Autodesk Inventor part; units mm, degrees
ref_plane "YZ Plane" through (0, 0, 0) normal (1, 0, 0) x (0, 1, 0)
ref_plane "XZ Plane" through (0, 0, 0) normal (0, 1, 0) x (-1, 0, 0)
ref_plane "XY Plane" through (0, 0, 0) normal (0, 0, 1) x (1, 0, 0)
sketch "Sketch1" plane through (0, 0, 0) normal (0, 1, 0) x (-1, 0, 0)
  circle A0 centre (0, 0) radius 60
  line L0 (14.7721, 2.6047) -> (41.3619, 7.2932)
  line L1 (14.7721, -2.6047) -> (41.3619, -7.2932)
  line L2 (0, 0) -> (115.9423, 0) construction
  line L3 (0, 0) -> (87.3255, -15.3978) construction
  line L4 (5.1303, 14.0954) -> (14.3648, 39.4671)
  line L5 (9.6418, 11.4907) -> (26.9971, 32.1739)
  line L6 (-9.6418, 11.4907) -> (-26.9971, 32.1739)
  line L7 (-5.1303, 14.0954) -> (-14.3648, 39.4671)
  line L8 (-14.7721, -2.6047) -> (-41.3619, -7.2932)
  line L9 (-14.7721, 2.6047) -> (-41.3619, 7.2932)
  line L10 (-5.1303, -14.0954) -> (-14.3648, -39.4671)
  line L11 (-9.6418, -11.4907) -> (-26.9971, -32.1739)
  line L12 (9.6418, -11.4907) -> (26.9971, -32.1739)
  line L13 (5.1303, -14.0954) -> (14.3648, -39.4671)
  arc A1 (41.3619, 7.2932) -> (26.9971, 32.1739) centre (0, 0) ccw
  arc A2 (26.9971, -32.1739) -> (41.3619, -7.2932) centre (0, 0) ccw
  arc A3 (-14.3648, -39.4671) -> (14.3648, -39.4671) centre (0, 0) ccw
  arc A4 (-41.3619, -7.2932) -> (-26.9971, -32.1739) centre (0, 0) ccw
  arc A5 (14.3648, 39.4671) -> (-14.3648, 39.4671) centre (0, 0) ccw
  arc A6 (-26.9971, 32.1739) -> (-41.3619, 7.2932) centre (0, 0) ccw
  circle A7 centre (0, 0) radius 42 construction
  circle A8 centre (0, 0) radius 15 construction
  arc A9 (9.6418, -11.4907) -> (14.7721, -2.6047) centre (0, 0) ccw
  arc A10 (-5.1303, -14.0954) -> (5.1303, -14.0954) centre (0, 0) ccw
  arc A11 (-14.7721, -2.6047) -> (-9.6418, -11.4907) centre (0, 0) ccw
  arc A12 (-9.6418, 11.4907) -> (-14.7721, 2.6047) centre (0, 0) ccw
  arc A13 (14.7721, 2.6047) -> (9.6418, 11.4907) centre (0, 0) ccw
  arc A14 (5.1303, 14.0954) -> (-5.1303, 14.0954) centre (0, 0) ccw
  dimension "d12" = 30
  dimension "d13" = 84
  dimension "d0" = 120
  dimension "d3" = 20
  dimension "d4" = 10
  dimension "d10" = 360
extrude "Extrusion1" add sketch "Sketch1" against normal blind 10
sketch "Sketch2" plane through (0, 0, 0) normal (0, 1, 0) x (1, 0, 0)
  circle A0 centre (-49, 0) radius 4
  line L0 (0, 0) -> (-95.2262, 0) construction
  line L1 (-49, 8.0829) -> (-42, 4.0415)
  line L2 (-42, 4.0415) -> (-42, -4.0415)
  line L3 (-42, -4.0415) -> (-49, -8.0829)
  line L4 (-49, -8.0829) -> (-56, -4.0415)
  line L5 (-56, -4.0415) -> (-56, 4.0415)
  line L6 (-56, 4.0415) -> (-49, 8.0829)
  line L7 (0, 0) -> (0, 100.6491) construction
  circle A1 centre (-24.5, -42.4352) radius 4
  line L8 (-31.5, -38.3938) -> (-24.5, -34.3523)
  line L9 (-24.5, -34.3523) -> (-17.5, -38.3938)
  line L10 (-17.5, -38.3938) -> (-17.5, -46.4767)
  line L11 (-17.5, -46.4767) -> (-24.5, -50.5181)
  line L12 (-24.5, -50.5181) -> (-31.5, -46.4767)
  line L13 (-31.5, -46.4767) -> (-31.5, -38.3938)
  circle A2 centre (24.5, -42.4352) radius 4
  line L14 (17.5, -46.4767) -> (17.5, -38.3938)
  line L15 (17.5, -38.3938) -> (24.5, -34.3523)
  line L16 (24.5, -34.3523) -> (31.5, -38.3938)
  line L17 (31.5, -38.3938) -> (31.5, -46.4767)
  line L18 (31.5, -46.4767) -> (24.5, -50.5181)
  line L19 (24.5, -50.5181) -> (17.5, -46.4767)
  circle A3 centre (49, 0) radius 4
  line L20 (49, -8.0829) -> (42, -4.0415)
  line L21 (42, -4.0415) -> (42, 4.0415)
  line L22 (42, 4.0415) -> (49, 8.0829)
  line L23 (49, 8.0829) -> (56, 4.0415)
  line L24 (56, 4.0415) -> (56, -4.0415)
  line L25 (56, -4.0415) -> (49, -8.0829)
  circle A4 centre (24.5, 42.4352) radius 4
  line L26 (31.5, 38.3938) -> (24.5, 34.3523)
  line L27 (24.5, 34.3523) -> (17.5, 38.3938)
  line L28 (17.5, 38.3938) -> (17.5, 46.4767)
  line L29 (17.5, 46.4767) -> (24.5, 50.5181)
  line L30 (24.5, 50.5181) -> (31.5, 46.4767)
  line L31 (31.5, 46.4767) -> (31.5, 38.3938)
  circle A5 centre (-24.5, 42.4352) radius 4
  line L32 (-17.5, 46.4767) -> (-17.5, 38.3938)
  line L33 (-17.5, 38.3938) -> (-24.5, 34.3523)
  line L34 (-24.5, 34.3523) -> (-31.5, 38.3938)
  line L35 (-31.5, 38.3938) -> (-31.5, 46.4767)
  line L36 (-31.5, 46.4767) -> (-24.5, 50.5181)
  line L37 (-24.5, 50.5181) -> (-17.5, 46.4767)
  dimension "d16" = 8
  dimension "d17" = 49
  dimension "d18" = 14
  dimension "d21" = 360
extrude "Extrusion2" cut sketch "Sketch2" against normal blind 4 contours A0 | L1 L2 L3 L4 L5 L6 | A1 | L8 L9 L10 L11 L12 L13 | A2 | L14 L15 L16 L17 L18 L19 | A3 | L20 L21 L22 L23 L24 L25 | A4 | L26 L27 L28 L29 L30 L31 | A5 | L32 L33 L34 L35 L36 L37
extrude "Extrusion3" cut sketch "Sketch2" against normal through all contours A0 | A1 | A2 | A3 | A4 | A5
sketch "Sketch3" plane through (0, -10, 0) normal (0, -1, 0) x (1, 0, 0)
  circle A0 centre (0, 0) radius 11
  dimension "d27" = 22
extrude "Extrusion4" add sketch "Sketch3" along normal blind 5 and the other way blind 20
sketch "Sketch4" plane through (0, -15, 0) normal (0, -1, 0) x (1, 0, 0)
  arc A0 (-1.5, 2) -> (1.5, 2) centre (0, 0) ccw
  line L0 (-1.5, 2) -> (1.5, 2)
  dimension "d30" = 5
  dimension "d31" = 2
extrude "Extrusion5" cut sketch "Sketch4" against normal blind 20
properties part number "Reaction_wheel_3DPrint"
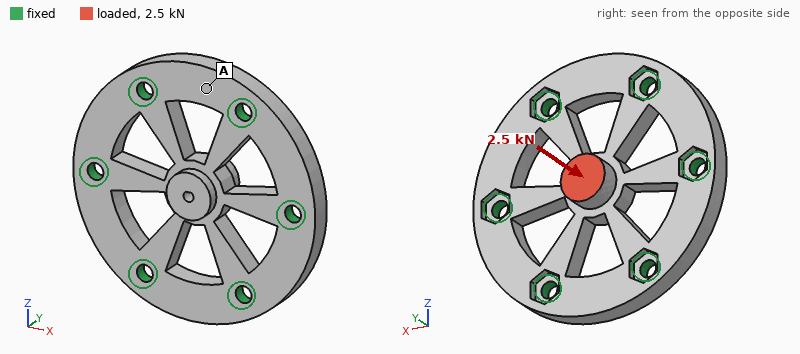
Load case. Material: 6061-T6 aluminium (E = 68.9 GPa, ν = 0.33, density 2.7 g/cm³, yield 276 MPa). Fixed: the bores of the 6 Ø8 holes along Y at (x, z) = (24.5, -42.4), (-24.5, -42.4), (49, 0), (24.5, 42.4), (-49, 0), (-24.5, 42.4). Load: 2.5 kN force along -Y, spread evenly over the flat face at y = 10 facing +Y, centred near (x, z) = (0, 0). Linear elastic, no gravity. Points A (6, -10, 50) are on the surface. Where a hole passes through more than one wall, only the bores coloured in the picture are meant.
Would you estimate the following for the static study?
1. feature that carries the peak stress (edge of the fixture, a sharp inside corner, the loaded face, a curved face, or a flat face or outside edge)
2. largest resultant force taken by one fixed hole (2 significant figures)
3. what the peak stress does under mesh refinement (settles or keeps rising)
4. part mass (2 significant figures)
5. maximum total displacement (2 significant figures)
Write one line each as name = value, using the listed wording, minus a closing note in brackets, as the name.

feature that carries the peak stress = edge of the fixture
largest resultant force taken by one fixed hole = 580 N
what the peak stress does under mesh refinement = keeps rising
part mass = 220 g
maximum total displacement = 49 µm
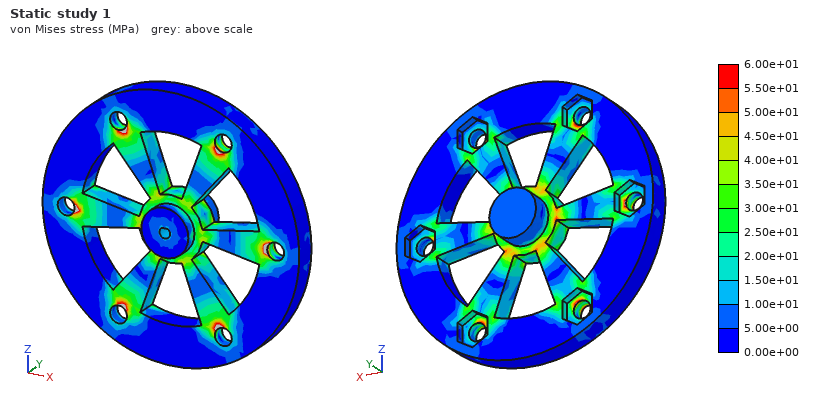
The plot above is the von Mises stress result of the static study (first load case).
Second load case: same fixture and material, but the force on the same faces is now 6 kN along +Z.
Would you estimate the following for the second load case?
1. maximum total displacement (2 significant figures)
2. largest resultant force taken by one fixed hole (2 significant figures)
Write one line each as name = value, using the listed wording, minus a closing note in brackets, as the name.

maximum total displacement = 83 µm
largest resultant force taken by one fixed hole = 1.9 kN
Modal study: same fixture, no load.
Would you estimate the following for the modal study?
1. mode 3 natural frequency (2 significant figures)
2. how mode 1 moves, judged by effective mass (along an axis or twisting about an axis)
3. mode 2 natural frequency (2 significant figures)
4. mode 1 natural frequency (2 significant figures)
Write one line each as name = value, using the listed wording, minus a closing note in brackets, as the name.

mode 3 natural frequency = 11 kHz
how mode 1 moves, judged by effective mass = along Y
mode 2 natural frequency = 11 kHz
mode 1 natural frequency = 5400 Hz
